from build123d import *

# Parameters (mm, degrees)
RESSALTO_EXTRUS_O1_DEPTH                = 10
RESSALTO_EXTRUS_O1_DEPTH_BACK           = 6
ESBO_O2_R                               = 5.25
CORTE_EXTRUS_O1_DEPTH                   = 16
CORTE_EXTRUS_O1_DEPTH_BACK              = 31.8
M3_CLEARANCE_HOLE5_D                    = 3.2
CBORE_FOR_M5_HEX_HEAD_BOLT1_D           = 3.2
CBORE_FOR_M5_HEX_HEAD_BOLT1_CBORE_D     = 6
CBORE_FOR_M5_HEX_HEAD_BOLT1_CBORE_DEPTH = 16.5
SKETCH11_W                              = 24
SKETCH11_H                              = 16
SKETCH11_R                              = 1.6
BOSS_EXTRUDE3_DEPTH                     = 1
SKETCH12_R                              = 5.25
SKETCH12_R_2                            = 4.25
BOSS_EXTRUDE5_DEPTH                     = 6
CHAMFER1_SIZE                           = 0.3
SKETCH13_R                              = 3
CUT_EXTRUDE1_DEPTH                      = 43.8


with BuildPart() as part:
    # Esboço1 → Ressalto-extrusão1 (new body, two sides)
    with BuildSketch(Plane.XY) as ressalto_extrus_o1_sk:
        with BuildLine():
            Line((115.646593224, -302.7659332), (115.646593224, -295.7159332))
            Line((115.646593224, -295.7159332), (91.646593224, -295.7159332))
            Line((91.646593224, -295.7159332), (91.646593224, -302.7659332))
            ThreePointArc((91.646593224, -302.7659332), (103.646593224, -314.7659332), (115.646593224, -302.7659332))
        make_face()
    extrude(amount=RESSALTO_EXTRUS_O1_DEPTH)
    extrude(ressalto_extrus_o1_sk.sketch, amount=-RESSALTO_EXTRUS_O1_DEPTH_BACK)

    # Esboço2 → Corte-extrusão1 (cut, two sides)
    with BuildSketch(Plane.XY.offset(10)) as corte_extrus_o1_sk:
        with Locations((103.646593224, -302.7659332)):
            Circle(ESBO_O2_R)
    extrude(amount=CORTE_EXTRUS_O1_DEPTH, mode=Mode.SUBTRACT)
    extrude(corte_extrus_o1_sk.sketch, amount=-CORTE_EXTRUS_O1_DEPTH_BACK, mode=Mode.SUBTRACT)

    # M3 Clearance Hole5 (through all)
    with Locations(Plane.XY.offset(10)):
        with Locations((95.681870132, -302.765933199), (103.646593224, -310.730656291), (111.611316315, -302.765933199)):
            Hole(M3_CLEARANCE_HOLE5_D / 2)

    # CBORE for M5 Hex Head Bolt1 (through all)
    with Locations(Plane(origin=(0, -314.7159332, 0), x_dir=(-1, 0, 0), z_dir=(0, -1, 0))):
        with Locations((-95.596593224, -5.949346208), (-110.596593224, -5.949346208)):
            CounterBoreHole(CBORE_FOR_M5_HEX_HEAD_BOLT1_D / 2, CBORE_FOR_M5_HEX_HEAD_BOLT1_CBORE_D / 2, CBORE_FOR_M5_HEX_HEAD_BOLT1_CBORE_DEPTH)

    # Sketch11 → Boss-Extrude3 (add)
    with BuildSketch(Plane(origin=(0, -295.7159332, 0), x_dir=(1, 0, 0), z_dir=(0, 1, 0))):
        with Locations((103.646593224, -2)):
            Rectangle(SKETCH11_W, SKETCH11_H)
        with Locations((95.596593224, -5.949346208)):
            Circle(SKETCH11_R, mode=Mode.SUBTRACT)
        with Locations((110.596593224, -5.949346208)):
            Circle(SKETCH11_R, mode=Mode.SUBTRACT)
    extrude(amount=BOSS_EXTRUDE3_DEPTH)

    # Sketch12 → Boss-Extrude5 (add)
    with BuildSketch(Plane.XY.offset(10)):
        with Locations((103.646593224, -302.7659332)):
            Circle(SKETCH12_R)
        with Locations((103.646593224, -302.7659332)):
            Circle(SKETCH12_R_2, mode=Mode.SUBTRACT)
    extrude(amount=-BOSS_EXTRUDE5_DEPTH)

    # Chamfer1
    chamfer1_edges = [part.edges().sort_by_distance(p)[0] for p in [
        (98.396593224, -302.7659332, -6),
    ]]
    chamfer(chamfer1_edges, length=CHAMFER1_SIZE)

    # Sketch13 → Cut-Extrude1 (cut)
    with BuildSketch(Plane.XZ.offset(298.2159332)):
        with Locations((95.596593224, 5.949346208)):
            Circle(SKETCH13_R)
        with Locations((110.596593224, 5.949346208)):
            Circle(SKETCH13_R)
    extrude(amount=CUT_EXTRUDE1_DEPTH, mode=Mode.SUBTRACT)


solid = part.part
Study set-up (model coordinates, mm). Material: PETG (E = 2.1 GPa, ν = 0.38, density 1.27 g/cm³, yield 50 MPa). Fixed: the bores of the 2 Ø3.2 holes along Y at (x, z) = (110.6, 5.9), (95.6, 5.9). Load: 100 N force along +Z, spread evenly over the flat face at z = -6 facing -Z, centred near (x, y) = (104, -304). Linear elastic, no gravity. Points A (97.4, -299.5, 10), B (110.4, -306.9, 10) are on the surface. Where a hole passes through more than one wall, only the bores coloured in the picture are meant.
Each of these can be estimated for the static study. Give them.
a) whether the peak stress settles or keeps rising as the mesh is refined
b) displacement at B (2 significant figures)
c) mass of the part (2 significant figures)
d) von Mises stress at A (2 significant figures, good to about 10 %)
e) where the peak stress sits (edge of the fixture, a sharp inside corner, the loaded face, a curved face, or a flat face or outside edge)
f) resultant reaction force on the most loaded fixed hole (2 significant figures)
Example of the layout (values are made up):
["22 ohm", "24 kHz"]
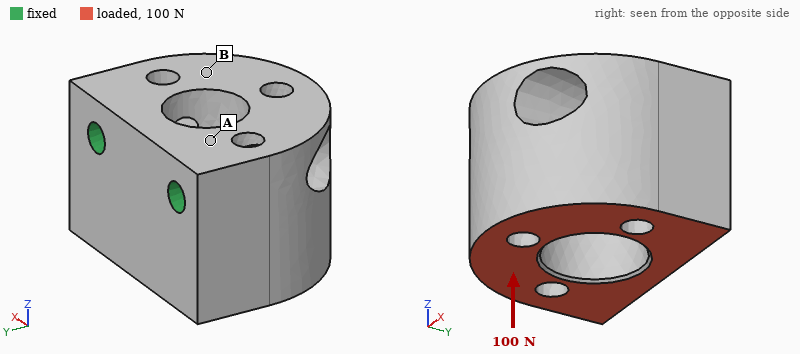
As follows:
["keeps rising", "0.076 mm", "5.6 g", "3.7 MPa", "edge of the fixture", "52 N"]
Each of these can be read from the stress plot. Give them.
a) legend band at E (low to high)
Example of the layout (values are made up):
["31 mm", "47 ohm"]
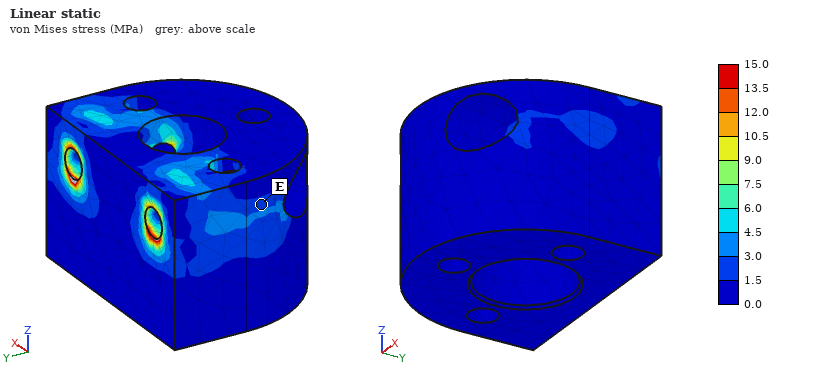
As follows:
["1.5 to 3.0 MPa"]
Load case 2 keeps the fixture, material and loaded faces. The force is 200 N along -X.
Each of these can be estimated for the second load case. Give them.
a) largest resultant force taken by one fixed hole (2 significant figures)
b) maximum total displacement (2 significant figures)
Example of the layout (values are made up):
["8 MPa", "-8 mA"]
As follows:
["180 N", "0.11 mm"]
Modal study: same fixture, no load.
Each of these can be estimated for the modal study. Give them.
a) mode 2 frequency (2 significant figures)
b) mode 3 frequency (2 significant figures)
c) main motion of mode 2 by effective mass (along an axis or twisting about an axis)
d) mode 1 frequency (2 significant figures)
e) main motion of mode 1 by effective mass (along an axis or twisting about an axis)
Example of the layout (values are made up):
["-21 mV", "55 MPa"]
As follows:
["3900 Hz", "6100 Hz", "along X", "2000 Hz", "along Z"]
